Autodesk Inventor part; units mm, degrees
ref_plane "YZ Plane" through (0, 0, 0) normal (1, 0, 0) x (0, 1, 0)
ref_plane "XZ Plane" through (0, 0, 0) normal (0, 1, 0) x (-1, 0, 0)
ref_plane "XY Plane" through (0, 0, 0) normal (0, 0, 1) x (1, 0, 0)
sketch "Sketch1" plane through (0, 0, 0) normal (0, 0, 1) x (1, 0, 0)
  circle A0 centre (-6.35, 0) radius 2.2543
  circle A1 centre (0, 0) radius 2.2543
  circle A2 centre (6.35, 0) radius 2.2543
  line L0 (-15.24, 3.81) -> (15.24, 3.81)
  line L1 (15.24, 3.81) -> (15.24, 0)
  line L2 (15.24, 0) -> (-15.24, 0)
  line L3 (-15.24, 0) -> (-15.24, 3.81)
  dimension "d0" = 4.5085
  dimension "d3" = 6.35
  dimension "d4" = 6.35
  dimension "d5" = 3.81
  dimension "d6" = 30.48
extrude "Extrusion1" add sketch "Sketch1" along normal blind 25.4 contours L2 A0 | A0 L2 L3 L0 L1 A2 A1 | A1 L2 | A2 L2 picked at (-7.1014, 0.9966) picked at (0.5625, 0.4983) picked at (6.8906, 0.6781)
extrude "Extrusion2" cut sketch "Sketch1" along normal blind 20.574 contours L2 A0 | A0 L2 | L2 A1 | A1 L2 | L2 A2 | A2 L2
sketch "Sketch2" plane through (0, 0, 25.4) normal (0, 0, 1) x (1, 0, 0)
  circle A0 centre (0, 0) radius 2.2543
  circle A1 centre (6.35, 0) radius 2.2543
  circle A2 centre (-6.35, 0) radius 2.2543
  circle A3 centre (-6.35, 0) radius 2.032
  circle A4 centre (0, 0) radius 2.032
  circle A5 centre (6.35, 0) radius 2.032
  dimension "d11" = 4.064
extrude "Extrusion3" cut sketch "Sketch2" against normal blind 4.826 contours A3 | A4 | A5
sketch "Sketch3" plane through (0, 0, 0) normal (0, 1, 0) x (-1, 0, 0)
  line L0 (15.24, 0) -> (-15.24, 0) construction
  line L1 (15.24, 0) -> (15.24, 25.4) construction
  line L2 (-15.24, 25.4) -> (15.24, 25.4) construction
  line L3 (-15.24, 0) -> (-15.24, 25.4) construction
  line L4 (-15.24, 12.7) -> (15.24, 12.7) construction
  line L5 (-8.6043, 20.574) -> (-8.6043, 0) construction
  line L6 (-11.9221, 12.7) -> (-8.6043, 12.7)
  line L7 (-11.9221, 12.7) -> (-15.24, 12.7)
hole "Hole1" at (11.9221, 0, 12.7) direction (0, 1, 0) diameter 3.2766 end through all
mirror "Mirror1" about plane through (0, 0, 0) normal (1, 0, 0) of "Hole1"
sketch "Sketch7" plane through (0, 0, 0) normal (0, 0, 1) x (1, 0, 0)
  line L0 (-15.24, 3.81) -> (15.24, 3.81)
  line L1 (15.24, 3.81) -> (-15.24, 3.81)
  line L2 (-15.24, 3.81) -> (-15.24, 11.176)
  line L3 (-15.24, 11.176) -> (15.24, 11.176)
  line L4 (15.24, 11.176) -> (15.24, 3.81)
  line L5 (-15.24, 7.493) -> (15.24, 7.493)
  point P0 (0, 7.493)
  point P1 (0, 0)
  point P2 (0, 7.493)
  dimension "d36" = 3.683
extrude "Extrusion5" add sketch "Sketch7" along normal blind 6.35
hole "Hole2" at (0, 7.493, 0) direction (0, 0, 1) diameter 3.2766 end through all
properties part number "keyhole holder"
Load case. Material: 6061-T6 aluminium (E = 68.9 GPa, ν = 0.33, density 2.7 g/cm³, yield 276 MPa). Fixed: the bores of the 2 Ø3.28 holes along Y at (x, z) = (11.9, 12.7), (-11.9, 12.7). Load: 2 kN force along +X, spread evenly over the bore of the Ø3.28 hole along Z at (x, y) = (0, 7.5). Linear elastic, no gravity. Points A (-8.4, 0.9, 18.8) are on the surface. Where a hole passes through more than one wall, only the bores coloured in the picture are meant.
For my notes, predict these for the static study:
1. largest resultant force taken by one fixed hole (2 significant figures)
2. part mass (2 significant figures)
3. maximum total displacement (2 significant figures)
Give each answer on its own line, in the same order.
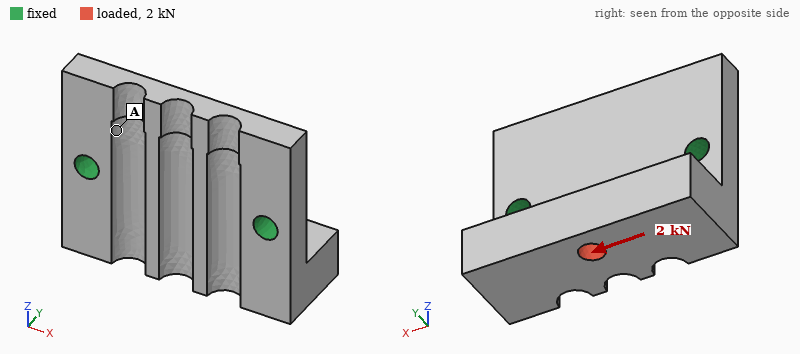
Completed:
1.3 kN
9.9 g
28 µm
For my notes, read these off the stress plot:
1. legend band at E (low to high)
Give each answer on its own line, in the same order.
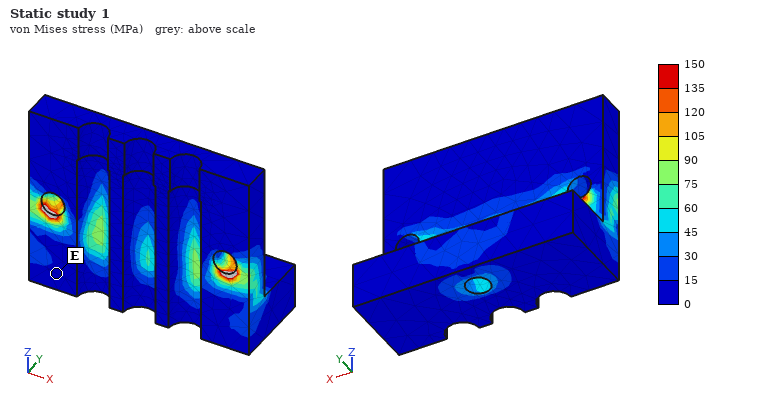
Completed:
0 to 15 MPa
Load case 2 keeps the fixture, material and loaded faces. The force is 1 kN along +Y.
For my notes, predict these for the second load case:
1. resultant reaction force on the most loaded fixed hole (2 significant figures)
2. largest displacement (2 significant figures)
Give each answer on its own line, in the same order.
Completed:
510 N
92 µm
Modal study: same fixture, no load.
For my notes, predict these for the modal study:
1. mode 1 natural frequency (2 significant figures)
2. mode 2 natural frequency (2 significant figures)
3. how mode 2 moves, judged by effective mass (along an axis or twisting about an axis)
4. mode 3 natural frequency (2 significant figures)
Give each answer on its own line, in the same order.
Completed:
8100 Hz
16 kHz
along Y
17 kHz
